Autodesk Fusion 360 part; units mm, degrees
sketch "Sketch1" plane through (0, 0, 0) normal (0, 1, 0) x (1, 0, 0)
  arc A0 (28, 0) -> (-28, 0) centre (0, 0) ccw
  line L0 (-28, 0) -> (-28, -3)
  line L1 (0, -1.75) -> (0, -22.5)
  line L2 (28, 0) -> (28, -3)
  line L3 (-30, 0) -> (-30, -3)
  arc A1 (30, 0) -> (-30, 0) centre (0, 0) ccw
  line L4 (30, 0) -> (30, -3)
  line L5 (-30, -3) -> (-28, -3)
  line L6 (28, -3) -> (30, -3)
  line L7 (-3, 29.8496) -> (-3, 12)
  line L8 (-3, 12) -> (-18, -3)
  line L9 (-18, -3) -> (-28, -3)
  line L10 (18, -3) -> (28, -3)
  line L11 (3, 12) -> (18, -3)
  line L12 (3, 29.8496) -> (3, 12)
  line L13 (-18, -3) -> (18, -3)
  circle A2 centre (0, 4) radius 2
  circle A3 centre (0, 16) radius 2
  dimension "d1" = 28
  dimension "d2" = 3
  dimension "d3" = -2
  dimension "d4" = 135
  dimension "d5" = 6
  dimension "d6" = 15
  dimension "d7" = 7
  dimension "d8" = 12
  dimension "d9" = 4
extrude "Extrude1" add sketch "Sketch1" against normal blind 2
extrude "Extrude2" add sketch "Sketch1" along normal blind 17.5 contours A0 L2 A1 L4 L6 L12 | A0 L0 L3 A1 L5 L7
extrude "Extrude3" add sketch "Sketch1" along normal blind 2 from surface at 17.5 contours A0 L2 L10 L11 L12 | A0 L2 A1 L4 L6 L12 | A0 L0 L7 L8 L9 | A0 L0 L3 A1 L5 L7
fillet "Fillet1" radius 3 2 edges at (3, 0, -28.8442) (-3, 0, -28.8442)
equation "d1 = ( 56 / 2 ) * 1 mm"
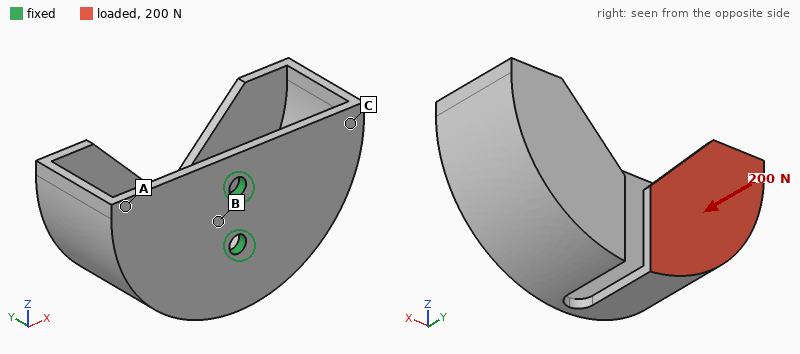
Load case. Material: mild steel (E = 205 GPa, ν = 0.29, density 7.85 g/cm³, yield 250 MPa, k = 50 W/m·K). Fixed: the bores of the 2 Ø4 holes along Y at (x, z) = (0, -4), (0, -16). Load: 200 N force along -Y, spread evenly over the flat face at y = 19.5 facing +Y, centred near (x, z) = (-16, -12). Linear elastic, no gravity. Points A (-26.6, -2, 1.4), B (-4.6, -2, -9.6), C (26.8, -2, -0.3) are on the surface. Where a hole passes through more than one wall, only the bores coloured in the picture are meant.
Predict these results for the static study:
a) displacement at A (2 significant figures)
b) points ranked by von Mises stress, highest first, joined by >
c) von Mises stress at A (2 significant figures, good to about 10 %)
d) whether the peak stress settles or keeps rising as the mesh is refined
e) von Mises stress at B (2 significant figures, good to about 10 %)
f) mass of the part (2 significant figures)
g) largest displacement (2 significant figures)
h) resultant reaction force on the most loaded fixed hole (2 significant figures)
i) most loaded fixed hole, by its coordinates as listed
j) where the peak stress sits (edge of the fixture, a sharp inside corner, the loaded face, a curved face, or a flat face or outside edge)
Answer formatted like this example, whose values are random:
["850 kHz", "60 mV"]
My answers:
["0.11 mm", "B > A > C", "43 MPa", "keeps rising", "93 MPa", "68 g", "0.14 mm", "130 N", "(0, -16)", "edge of the fixture"]
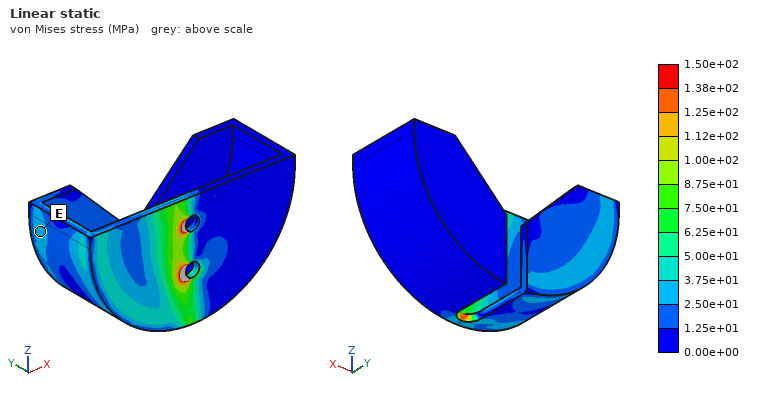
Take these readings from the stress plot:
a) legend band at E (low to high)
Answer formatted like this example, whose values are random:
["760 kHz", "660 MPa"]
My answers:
["2.50e+01 to 3.75e+01 MPa"]
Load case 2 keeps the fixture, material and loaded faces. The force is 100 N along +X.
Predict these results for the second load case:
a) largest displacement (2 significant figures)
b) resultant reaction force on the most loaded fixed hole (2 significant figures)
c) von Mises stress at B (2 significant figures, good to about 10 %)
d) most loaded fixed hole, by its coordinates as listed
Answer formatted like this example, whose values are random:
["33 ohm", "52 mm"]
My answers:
["0.17 mm", "67 N", "64 MPa", "(0, -16)"]
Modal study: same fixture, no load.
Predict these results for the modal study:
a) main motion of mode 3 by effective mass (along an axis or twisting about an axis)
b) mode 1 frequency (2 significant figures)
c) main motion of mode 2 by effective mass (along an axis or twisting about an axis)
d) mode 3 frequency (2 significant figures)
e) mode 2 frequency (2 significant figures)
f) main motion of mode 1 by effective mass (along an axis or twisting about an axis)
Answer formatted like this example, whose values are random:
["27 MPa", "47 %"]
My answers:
["along Z", "920 Hz", "along Y", "1300 Hz", "1100 Hz", "along X"]
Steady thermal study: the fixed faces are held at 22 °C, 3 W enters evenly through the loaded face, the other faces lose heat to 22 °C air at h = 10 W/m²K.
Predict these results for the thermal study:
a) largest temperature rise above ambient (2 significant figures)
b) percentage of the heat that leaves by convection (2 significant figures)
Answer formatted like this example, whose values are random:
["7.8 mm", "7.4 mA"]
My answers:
["29 K", "23 %"]
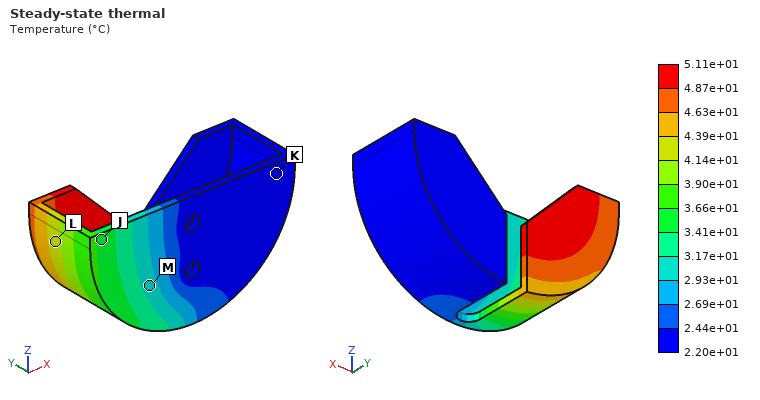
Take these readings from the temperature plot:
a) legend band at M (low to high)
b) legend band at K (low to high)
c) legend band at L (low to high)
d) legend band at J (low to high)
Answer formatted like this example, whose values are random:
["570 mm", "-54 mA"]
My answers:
["2.93e+01 to 3.17e+01 °C", "2.20e+01 to 2.44e+01 °C", "4.14e+01 to 4.39e+01 °C", "3.41e+01 to 3.66e+01 °C"]
